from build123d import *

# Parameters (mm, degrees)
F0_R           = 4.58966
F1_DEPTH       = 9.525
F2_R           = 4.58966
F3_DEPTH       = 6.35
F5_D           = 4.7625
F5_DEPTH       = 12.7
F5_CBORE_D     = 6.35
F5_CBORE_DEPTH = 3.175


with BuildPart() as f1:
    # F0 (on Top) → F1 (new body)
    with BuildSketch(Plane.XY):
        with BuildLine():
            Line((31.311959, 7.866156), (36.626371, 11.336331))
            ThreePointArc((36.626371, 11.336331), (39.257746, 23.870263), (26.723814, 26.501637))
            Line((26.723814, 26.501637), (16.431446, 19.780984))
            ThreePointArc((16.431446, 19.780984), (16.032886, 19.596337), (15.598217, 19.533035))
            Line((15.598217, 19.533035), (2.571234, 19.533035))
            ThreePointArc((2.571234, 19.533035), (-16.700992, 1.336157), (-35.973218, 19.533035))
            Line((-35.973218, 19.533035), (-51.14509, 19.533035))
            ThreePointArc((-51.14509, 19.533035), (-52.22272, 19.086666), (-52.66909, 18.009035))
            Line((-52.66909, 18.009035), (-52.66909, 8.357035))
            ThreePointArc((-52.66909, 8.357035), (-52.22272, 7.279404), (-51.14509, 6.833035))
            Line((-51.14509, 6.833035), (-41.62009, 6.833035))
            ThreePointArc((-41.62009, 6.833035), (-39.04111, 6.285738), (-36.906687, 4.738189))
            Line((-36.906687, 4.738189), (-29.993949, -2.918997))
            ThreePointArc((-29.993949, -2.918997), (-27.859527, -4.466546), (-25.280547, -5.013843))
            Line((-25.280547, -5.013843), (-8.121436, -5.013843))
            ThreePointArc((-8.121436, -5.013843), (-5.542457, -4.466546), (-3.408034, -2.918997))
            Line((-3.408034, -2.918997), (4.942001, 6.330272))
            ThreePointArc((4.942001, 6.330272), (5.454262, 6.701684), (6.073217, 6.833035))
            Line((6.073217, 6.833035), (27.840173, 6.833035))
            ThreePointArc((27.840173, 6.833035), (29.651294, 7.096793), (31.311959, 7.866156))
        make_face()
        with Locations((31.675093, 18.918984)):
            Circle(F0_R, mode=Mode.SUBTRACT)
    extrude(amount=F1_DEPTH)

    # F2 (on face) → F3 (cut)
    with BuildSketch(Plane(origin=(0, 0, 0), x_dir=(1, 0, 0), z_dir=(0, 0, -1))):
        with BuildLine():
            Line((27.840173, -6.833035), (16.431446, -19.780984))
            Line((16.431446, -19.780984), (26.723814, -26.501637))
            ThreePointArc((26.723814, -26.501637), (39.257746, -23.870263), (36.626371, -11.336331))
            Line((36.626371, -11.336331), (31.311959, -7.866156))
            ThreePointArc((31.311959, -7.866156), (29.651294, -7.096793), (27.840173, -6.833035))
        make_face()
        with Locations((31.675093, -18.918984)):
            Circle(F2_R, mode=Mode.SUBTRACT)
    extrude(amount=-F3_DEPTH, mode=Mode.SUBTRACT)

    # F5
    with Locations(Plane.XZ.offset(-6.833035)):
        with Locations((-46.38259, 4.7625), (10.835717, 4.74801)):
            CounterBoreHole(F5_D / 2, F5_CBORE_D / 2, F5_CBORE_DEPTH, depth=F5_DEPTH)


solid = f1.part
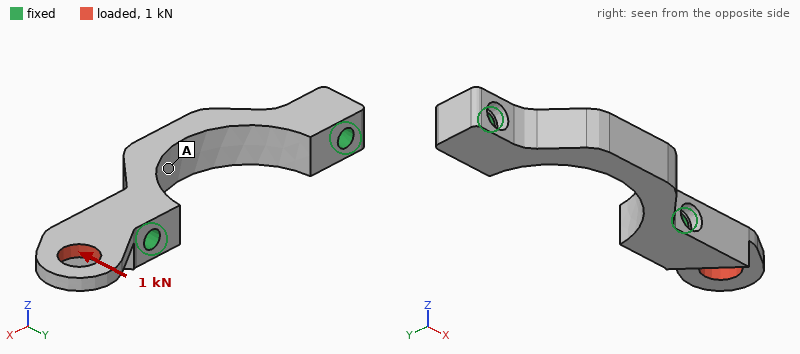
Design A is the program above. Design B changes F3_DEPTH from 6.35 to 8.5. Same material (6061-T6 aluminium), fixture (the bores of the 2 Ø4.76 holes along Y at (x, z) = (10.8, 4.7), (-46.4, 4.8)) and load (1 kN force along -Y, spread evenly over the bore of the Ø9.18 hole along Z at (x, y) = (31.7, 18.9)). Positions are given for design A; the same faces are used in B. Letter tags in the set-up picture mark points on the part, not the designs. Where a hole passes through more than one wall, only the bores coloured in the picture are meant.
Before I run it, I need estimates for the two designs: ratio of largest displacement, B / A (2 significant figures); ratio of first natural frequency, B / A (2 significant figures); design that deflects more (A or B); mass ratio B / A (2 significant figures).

2.0
0.41
B
0.93
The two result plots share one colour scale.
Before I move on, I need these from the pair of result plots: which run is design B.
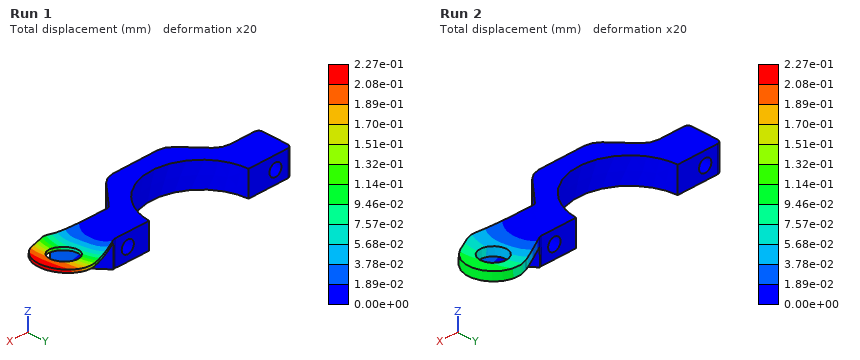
Run 1
